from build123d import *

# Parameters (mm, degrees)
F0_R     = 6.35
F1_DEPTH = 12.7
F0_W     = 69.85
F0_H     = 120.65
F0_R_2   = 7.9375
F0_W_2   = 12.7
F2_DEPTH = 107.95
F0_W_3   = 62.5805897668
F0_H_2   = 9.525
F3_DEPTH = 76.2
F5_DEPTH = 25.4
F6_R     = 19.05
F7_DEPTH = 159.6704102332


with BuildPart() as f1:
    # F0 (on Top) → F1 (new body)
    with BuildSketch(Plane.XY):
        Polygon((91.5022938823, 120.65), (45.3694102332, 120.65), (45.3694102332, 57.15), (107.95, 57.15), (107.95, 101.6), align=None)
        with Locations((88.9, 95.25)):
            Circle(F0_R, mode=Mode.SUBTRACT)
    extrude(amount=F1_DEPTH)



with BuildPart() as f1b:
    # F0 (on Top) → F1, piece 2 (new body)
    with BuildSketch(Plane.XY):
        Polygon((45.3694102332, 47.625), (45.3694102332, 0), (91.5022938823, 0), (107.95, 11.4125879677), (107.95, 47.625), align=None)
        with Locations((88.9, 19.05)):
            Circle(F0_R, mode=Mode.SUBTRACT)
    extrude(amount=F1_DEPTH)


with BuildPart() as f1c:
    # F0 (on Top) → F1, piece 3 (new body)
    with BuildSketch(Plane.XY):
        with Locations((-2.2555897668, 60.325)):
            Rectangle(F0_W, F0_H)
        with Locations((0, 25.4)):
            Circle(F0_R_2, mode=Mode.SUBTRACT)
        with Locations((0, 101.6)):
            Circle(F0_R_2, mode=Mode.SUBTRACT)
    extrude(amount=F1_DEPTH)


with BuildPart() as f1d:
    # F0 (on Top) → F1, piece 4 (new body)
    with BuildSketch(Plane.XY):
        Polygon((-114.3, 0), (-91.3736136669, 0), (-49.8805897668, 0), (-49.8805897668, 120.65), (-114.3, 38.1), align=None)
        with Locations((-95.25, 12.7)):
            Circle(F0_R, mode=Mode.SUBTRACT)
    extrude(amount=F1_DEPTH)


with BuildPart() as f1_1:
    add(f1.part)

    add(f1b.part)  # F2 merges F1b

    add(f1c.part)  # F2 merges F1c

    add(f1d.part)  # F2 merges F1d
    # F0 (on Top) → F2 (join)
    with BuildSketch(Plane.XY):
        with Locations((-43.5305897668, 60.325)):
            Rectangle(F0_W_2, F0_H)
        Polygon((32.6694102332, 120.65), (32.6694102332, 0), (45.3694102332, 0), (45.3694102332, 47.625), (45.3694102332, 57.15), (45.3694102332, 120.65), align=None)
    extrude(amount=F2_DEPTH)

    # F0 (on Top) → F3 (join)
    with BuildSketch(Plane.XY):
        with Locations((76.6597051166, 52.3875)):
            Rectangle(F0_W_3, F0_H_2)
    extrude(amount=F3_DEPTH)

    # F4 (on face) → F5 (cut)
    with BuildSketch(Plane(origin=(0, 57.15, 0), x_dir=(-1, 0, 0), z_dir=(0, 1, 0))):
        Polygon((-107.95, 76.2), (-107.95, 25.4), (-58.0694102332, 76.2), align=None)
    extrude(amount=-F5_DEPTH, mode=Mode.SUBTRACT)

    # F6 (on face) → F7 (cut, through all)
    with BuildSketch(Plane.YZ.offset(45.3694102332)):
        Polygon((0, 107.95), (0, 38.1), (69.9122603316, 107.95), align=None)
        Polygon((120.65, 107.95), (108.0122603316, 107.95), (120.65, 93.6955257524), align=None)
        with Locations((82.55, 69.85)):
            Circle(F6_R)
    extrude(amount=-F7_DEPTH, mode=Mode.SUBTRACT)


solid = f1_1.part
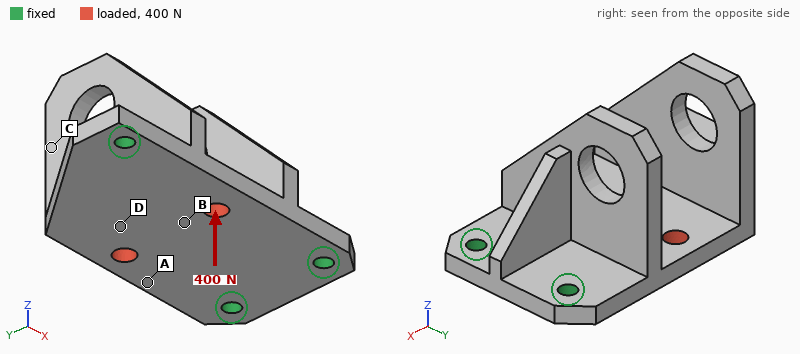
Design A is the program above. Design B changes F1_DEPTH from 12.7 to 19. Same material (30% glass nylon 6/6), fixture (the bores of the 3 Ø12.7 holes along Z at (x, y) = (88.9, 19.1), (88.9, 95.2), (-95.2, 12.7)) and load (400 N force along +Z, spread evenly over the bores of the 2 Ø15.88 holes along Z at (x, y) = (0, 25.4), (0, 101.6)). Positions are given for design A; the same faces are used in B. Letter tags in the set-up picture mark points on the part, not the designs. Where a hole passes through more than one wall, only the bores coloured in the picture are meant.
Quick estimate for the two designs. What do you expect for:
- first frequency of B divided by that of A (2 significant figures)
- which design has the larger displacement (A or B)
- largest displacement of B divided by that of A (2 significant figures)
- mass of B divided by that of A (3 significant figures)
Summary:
1.5
A
0.36
1.24
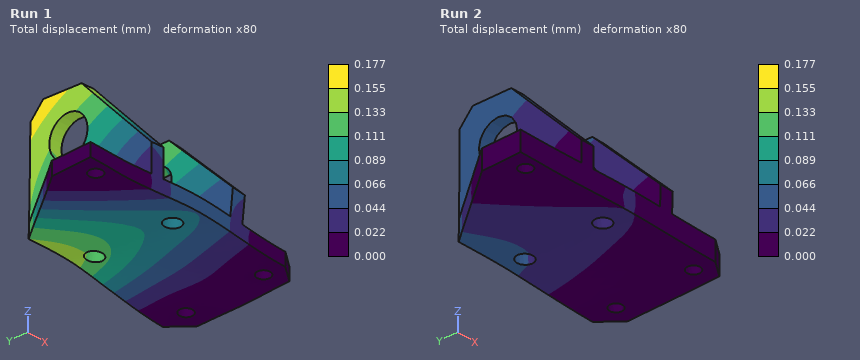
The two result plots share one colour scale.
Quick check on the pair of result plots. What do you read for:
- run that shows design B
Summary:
Run 2
